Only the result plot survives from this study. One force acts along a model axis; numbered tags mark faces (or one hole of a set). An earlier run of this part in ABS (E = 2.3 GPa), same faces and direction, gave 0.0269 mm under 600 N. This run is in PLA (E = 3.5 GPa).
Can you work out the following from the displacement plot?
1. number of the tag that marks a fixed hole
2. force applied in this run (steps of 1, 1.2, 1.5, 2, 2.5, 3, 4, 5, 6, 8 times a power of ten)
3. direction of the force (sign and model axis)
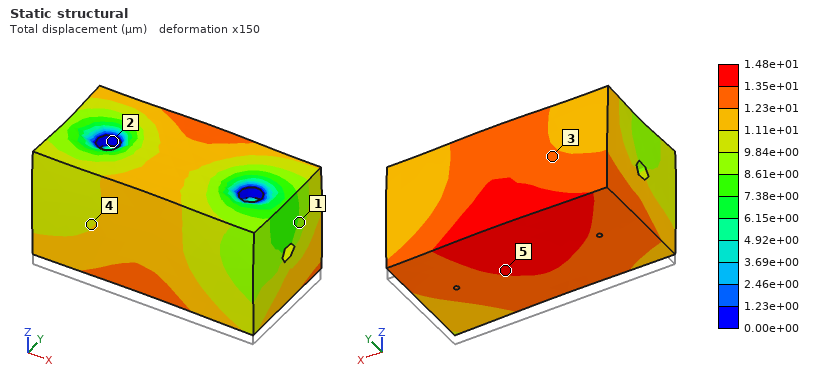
2
500 N
+Z
